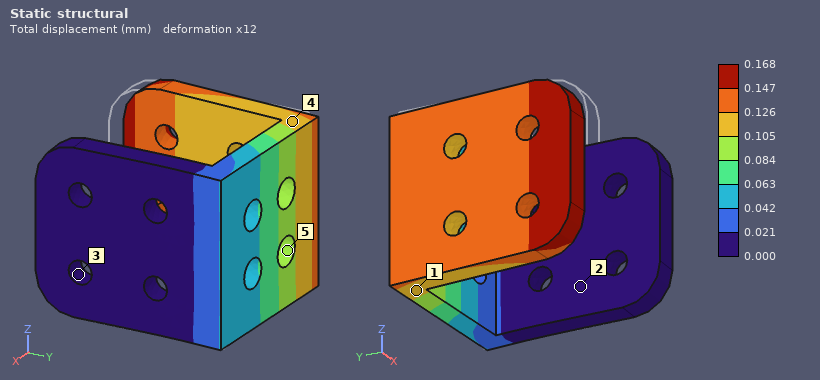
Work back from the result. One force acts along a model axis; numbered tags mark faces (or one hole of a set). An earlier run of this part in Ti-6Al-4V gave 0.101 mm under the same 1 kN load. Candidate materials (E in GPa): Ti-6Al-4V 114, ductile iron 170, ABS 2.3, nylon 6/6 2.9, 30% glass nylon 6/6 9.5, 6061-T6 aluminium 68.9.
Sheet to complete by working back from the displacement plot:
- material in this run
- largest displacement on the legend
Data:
6061-T6 aluminium
0.168 mm
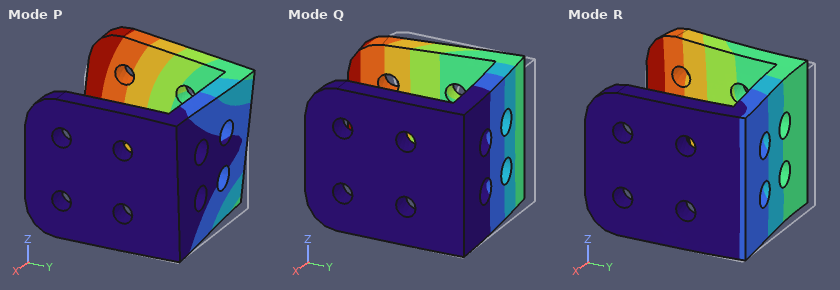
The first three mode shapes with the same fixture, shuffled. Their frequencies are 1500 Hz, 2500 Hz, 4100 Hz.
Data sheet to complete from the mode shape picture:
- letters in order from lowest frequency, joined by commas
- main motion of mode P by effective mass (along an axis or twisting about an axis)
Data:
Q, P, R
along Z
